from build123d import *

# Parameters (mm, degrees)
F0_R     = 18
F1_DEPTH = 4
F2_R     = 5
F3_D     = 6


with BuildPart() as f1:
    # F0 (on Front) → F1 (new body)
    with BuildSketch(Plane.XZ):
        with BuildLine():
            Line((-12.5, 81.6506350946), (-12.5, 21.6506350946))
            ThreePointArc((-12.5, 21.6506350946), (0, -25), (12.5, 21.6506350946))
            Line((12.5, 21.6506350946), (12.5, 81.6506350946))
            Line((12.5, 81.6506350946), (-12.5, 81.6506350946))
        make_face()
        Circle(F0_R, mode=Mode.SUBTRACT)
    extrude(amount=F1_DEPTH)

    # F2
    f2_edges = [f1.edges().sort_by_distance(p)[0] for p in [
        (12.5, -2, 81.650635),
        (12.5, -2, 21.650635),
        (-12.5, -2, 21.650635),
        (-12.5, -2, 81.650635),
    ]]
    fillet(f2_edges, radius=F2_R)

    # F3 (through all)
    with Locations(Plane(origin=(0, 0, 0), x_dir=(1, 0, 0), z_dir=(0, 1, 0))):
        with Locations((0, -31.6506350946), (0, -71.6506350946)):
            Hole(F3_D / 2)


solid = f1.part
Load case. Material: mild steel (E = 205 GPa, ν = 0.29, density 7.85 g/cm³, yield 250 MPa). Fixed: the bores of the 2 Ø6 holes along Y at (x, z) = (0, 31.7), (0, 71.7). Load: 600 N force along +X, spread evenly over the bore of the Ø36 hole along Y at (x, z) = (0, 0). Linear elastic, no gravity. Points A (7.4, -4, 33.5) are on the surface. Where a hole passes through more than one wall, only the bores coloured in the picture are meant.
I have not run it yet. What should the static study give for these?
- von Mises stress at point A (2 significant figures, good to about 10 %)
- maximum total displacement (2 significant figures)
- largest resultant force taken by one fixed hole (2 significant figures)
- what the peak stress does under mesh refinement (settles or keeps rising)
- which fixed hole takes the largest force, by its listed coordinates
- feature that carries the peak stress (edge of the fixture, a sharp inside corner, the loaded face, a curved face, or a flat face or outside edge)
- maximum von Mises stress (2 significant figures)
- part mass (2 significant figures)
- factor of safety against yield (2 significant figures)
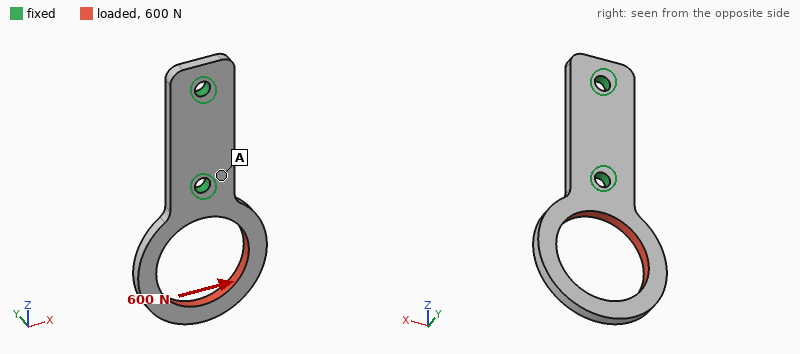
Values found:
21 MPa
89 µm
900 N
settles
(0, 31.7)
a curved face
140 MPa
73 g
1.7
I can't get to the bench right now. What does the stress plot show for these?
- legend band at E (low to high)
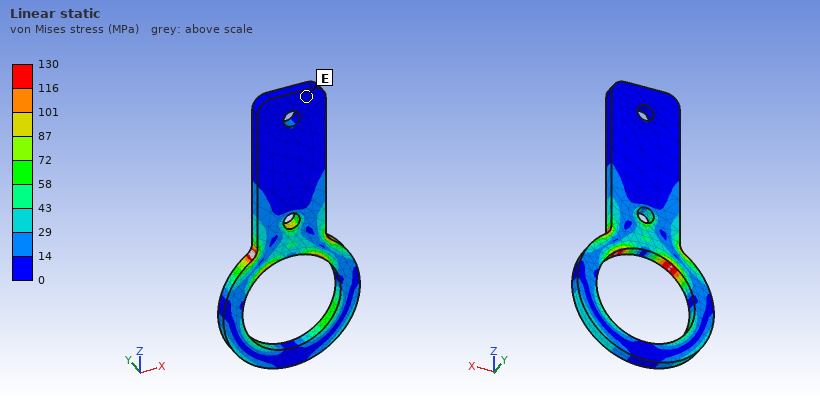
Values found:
0 to 14 MPa
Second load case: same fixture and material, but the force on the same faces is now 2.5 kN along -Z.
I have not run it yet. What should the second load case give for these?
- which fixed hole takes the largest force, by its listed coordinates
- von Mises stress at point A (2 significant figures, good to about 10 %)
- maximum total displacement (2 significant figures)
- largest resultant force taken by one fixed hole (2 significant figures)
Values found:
(0, 31.7)
23 MPa
46 µm
2.1 kN
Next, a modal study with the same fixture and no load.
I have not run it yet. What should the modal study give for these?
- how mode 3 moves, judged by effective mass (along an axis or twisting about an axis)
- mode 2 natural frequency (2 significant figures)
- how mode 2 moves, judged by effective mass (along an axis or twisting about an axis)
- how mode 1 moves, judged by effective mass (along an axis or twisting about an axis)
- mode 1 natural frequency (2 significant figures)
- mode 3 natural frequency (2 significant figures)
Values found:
along X
2000 Hz
twisting about Z
along Y
920 Hz
2600 Hz
